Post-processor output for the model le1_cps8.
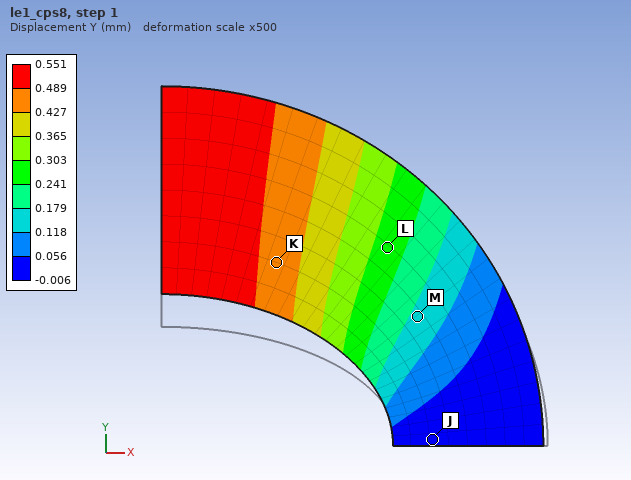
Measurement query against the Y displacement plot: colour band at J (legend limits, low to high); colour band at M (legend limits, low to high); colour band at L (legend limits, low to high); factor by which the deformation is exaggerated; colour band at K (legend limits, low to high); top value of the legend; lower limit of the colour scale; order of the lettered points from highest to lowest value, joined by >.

-0.006 to 0.056 mm
0.118 to 0.179 mm
0.241 to 0.303 mm
500
0.427 to 0.489 mm
0.551 mm
-0.006 mm
K > L > M > J
